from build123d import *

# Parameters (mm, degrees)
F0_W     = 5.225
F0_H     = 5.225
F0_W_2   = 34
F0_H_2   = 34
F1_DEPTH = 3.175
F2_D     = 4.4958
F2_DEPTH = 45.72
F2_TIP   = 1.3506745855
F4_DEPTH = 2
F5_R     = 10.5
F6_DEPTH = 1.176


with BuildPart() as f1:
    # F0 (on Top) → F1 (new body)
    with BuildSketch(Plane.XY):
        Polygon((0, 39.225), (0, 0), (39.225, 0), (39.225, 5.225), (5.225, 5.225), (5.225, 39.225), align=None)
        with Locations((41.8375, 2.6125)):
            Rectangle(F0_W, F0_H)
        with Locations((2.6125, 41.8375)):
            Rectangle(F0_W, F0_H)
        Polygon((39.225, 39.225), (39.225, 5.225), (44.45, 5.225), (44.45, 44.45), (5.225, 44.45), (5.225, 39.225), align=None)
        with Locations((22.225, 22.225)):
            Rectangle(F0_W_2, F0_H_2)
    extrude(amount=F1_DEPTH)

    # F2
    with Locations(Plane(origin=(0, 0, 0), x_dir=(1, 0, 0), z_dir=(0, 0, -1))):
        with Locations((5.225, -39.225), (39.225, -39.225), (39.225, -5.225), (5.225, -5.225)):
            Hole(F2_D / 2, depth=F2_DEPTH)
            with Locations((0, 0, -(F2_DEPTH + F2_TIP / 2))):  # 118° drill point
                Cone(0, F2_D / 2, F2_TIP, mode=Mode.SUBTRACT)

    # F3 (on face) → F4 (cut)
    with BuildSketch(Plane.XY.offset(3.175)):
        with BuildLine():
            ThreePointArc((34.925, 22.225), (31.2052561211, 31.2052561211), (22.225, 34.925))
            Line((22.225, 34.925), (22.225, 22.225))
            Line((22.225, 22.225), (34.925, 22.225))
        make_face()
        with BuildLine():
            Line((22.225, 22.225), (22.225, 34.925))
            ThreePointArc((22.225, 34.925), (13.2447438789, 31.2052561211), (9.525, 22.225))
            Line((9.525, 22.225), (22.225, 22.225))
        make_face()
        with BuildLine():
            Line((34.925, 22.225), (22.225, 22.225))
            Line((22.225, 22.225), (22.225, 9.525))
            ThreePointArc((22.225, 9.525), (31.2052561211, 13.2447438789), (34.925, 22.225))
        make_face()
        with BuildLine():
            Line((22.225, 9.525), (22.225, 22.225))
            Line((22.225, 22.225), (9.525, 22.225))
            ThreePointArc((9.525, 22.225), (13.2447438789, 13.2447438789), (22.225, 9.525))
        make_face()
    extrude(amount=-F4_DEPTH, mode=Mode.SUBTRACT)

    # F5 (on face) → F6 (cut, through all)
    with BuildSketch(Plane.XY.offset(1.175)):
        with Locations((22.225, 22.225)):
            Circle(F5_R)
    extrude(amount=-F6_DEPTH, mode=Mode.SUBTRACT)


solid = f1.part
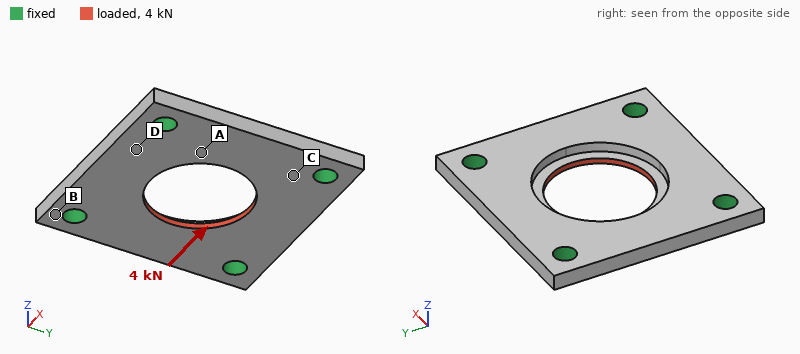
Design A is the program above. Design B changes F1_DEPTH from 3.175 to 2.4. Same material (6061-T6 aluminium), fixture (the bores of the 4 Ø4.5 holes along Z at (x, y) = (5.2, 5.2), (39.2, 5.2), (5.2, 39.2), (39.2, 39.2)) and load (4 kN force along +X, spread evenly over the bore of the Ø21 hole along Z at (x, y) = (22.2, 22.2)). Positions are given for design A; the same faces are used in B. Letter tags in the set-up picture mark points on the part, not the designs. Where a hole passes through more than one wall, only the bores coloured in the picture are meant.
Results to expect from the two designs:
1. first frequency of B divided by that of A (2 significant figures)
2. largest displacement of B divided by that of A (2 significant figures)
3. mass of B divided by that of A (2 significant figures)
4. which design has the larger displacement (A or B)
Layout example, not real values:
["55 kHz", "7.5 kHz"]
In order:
["0.78", "1.2", "0.77", "B"]
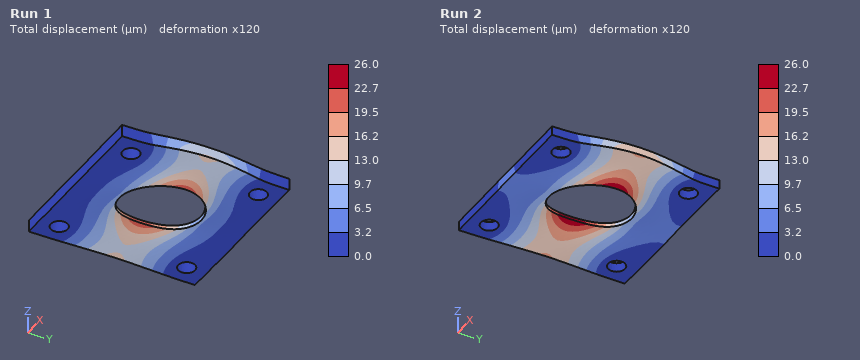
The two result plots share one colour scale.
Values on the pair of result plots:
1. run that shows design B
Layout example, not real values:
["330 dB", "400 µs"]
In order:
["Run 2"]
